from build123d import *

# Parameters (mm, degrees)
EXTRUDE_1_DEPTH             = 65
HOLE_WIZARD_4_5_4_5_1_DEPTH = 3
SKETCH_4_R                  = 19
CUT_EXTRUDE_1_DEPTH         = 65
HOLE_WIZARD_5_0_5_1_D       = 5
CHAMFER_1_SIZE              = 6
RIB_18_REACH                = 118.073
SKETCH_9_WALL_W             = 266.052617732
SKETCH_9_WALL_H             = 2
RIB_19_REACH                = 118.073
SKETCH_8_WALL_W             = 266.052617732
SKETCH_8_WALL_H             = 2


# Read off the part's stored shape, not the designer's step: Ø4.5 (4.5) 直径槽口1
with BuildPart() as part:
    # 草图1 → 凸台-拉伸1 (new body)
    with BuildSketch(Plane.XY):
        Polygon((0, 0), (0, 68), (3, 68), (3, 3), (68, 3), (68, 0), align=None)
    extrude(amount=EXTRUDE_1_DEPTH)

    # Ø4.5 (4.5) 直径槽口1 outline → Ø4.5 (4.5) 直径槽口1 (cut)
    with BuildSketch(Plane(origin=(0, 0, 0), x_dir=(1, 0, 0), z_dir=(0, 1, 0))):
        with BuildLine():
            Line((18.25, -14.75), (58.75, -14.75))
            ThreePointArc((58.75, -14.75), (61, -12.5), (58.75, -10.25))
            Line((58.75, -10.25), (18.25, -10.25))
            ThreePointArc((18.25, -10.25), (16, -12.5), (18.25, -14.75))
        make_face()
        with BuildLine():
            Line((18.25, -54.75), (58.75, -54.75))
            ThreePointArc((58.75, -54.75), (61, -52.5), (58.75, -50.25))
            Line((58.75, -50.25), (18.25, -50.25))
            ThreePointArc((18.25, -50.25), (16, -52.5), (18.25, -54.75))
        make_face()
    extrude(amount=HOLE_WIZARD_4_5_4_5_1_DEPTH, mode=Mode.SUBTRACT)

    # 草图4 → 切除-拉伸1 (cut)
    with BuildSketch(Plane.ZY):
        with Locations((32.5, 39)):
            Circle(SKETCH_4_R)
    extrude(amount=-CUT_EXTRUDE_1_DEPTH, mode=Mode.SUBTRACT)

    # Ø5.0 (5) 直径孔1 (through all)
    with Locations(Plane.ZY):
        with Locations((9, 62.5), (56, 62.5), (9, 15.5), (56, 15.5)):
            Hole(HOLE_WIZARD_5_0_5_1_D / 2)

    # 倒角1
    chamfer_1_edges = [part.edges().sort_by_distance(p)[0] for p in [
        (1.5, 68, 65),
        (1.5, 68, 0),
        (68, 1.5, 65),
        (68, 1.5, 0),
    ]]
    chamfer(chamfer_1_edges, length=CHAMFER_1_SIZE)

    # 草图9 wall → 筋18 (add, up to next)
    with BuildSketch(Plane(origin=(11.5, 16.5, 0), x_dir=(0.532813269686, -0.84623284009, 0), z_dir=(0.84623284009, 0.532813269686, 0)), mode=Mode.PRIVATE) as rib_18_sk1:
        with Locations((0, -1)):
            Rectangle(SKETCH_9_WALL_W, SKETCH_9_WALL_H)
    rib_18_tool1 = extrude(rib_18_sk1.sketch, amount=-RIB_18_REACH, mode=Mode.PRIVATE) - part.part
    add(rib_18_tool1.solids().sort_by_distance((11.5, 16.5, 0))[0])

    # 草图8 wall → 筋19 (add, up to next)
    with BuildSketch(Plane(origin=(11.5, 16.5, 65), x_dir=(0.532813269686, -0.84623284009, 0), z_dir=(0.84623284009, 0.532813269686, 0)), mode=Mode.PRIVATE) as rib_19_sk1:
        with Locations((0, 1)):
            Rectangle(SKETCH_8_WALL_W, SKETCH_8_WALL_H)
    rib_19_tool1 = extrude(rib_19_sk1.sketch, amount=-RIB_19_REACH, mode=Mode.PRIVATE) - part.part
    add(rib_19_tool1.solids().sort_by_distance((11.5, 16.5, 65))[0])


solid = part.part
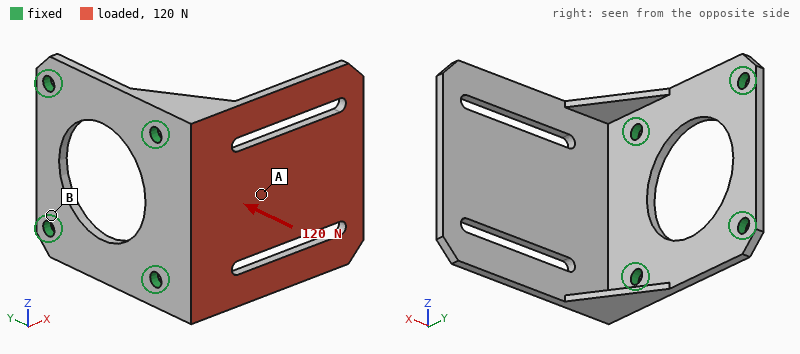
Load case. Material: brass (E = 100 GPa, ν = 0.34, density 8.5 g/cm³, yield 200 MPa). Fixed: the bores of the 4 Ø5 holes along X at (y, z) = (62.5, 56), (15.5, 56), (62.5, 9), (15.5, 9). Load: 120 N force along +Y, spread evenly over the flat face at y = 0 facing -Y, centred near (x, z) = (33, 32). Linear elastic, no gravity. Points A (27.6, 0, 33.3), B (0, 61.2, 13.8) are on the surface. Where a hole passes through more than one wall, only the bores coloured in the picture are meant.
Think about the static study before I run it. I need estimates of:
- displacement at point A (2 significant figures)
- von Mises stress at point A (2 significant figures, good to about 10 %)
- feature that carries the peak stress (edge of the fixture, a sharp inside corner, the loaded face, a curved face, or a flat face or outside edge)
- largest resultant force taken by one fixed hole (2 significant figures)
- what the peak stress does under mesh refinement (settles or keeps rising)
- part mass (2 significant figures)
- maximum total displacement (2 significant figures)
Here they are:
0.080 mm
12 MPa
edge of the fixture
63 N
keeps rising
190 g
0.29 mm
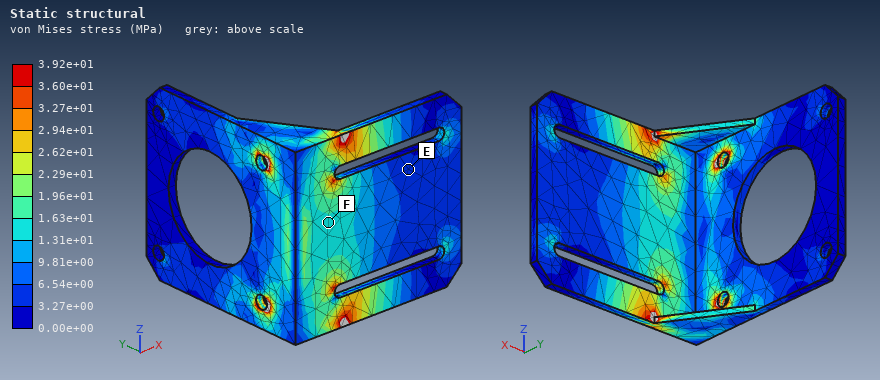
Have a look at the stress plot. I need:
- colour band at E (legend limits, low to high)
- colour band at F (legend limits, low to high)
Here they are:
3.27e+00 to 6.54e+00 MPa
1.31e+01 to 1.63e+01 MPa
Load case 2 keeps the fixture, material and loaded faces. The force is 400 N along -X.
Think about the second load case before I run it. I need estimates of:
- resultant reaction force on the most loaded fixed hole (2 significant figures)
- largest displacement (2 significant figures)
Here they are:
220 N
0.15 mm
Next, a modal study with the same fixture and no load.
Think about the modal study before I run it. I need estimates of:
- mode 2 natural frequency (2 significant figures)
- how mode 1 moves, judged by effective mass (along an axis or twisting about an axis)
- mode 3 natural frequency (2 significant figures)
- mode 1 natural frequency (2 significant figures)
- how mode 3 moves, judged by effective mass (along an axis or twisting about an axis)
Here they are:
1000 Hz
along Y
1700 Hz
400 Hz
along Z
